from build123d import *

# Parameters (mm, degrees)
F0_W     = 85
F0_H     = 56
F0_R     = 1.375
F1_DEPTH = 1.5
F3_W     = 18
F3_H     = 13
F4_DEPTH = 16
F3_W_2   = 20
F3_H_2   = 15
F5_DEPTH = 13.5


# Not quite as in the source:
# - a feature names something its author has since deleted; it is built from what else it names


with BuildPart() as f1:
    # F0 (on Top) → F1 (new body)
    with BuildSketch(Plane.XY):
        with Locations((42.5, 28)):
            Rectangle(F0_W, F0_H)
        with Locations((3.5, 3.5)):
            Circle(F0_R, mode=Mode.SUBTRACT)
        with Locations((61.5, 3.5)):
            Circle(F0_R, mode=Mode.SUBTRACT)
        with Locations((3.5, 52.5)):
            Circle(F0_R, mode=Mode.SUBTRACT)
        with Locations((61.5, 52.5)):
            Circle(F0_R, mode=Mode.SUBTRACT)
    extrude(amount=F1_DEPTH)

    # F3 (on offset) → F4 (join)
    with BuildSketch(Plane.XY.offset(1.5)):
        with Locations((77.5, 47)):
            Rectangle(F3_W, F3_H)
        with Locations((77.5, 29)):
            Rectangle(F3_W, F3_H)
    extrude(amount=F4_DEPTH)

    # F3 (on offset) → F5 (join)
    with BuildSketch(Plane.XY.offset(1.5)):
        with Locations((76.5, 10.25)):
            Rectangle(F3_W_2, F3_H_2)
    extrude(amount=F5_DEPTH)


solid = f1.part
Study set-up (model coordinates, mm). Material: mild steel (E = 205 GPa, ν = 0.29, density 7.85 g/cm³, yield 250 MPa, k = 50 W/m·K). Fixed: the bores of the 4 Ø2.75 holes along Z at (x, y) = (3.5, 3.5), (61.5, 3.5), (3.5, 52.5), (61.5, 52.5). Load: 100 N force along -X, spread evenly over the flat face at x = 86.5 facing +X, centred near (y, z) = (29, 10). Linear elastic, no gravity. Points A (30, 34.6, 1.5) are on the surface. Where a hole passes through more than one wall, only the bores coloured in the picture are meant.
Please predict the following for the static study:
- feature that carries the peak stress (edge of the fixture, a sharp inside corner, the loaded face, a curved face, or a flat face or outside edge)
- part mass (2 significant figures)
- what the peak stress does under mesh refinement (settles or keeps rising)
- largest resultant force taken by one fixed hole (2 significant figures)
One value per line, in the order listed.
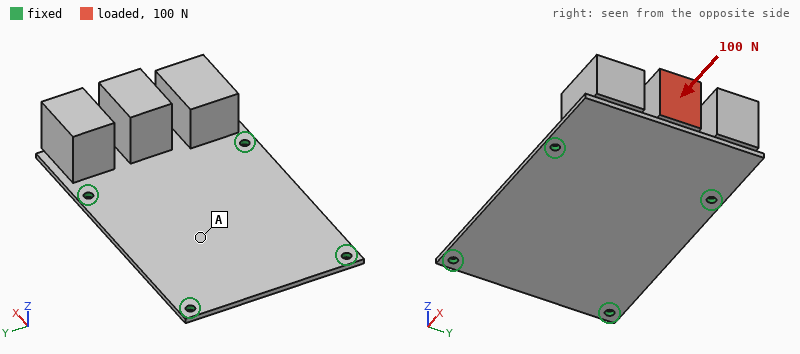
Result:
edge of the fixture
150 g
keeps rising
41 N
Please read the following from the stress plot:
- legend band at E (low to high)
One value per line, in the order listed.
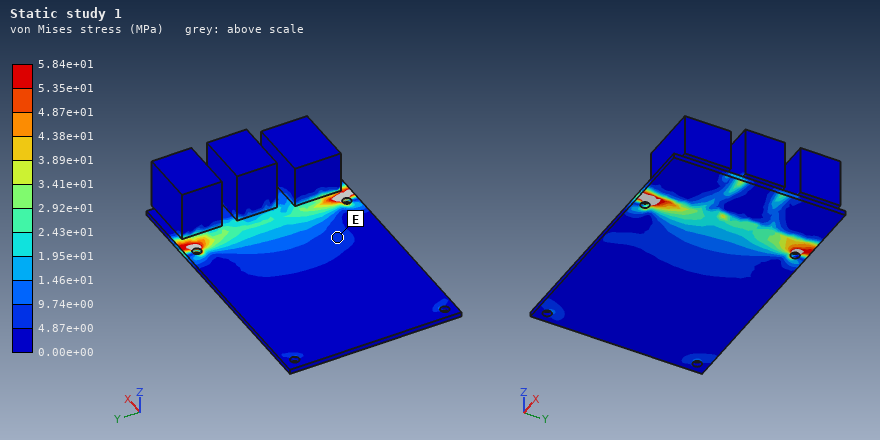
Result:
4.87e+00 to 9.74e+00 MPa
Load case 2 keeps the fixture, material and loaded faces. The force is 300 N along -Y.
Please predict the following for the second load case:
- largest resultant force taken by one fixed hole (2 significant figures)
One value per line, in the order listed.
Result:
220 N
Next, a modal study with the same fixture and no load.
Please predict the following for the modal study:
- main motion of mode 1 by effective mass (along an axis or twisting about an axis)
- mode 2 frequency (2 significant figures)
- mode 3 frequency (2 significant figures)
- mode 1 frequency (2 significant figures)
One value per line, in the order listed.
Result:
along Z
1600 Hz
1900 Hz
520 Hz
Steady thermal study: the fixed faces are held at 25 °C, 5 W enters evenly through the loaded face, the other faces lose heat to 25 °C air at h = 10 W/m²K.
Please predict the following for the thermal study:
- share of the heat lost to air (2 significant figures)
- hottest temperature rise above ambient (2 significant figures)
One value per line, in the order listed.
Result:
25 %
31 K
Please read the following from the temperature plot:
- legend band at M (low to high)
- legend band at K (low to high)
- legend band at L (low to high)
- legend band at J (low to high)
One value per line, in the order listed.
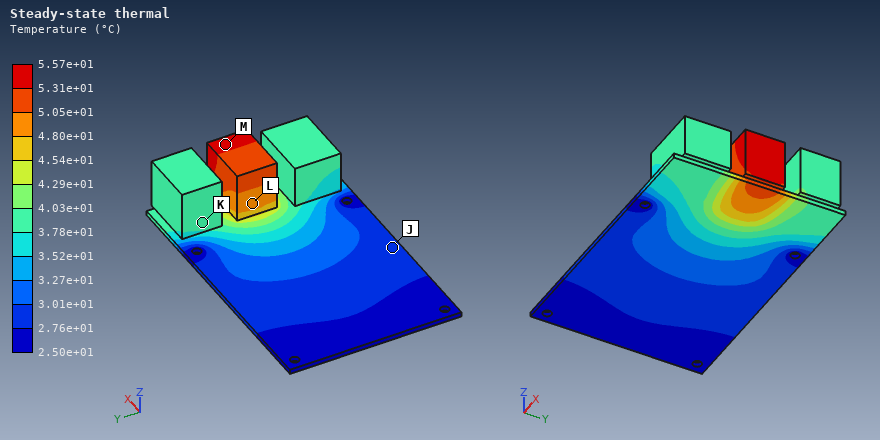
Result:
5.31e+01 to 5.57e+01 °C
3.78e+01 to 4.03e+01 °C
4.80e+01 to 5.05e+01 °C
2.76e+01 to 3.01e+01 °C
